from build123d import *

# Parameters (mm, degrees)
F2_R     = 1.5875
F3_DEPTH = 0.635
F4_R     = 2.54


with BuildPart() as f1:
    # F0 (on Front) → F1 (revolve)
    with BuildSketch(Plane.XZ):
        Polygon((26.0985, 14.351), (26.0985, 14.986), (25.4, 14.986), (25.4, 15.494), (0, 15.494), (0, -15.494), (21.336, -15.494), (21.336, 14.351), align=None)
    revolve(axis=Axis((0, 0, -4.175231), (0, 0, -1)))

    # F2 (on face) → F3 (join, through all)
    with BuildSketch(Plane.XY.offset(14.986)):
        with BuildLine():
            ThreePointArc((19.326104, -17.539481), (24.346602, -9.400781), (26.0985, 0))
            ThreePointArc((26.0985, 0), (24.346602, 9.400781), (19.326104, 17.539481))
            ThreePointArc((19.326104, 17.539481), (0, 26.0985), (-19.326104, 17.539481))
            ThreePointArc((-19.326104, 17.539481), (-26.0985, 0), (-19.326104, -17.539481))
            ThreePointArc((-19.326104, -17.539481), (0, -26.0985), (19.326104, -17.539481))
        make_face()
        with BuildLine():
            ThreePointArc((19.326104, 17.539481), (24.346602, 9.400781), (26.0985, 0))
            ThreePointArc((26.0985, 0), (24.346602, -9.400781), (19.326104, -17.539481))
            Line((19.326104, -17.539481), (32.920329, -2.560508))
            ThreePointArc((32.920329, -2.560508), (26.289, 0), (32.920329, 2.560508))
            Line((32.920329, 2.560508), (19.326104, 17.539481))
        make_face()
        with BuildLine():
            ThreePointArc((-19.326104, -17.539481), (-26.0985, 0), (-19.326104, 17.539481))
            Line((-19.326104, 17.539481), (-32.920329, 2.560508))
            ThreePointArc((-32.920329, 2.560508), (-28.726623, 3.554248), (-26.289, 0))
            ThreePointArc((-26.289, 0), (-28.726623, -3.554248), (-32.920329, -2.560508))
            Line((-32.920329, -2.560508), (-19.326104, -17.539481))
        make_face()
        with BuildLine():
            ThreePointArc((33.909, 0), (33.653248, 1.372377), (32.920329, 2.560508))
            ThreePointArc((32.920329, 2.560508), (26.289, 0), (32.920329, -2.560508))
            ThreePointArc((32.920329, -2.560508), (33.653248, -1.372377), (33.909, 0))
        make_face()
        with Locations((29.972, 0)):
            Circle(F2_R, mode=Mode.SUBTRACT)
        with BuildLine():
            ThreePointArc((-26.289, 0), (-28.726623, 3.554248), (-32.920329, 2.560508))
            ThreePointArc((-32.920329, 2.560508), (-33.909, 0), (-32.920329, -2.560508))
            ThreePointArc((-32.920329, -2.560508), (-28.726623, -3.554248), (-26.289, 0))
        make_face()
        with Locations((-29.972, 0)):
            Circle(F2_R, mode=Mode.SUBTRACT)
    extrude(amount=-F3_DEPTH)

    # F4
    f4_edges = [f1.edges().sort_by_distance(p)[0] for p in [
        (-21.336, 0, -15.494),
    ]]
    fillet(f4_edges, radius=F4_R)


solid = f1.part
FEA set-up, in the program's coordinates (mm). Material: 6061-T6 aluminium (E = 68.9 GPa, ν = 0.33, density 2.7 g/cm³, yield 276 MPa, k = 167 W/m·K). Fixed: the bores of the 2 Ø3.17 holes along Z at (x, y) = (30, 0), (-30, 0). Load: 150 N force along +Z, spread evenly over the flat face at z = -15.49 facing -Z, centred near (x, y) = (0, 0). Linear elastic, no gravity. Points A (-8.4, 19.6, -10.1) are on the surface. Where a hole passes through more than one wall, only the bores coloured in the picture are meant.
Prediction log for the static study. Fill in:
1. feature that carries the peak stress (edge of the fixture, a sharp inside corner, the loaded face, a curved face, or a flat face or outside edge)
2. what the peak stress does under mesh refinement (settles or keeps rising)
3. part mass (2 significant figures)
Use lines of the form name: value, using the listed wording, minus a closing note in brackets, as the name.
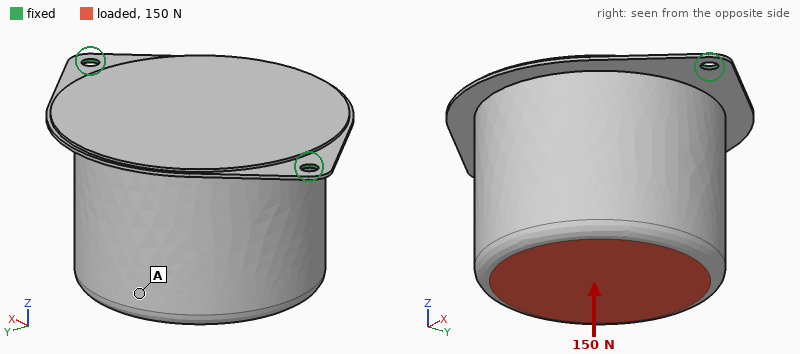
feature that carries the peak stress: edge of the fixture
what the peak stress does under mesh refinement: keeps rising
part mass: 120 g
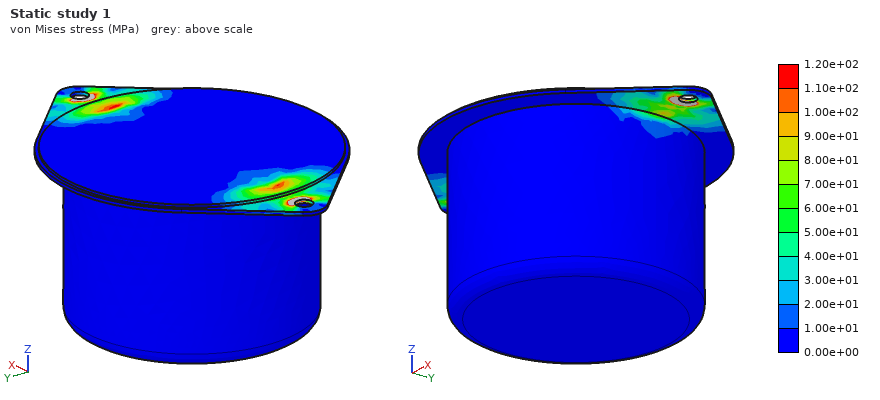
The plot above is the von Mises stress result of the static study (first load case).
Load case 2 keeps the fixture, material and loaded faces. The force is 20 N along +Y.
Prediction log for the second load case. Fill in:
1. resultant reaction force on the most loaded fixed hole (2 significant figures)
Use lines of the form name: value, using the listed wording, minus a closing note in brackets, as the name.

resultant reaction force on the most loaded fixed hole: 10 N
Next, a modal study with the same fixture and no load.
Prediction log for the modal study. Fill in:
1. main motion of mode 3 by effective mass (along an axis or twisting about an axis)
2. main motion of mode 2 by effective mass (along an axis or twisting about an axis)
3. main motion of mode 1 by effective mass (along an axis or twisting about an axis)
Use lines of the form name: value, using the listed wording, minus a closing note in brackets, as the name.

main motion of mode 3 by effective mass: along X
main motion of mode 2 by effective mass: along Z
main motion of mode 1 by effective mass: along Y
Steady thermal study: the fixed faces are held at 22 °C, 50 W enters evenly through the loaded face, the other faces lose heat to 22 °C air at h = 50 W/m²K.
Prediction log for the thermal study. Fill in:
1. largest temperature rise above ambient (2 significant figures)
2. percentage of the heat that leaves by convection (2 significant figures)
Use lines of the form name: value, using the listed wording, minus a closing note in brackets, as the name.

largest temperature rise above ambient: 74 K
percentage of the heat that leaves by convection: 50 %
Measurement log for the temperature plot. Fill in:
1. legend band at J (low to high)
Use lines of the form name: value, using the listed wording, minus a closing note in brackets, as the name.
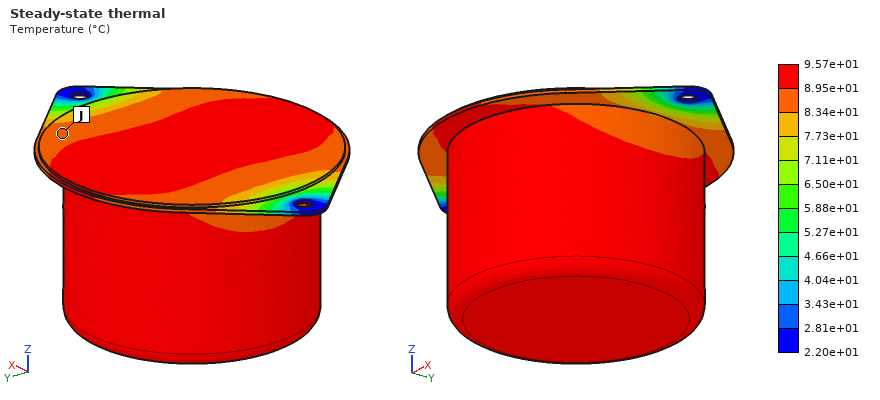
legend band at J: 8.34e+01 to 8.95e+01 °C
